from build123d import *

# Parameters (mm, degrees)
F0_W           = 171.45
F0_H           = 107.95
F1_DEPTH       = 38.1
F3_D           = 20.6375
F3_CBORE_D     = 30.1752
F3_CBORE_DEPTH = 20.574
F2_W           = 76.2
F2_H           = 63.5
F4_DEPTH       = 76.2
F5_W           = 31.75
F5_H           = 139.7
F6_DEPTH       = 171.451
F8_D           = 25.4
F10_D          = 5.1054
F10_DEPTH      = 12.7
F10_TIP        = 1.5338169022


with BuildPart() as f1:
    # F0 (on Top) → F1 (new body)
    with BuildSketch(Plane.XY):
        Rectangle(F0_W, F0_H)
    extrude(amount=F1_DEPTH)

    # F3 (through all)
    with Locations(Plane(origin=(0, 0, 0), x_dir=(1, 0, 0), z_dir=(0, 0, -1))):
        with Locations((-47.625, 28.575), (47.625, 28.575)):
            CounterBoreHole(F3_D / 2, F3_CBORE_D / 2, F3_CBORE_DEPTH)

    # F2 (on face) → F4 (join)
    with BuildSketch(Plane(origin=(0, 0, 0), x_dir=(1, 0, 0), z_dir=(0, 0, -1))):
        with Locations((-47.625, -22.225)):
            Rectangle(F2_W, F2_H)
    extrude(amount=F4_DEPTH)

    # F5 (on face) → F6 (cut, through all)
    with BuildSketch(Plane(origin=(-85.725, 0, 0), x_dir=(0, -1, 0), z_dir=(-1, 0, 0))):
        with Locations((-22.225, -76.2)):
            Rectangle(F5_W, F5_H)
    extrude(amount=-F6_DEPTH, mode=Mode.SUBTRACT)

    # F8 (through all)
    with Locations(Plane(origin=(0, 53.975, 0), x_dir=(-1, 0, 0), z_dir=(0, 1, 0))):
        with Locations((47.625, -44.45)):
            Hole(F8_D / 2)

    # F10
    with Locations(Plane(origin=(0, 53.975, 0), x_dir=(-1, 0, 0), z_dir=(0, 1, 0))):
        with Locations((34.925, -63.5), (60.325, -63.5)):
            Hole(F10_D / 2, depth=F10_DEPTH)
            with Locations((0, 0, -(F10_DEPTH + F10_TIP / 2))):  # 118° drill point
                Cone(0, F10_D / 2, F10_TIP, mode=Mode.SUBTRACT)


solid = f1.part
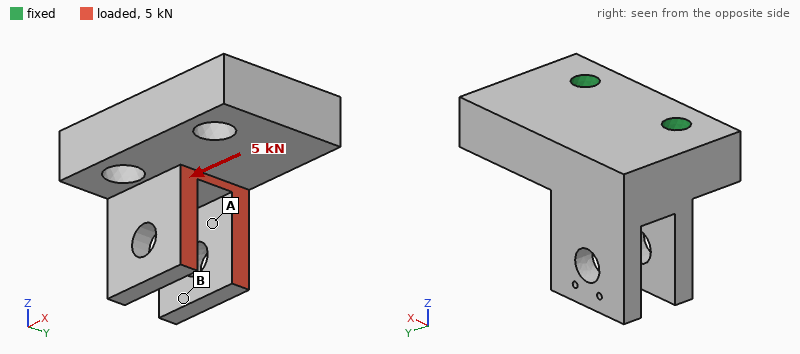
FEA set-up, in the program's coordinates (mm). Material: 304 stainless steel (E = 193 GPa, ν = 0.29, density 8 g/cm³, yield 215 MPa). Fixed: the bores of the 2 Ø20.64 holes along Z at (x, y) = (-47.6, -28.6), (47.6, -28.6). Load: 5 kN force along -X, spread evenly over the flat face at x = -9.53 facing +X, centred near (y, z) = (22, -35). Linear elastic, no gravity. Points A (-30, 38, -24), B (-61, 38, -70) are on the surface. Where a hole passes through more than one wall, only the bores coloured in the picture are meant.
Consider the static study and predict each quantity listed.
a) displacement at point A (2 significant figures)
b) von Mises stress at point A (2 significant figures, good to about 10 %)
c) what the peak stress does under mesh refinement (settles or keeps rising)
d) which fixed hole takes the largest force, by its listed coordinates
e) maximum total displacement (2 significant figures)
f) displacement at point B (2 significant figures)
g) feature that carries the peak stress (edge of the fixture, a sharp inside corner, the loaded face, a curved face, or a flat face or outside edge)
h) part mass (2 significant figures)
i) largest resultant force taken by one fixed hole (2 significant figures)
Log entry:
5.9 µm
3.8 MPa
keeps rising
(47.6, -28.6)
15 µm
13 µm
edge of the fixture
6.8 kg
5.1 kN
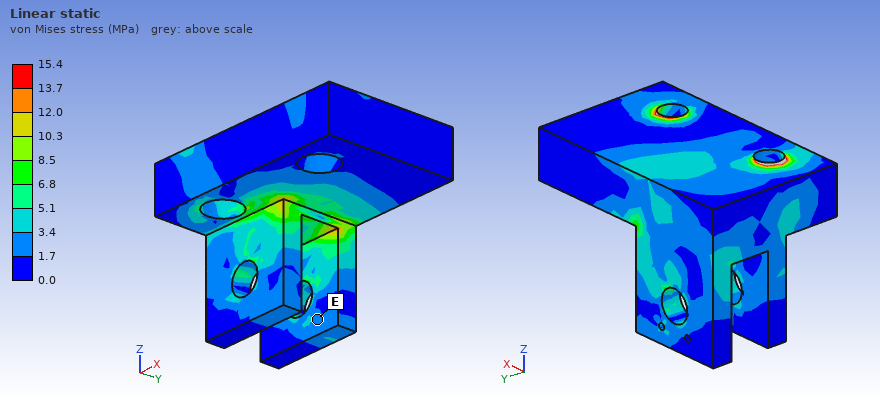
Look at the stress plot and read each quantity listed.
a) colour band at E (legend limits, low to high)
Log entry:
1.7 to 3.4 MPa
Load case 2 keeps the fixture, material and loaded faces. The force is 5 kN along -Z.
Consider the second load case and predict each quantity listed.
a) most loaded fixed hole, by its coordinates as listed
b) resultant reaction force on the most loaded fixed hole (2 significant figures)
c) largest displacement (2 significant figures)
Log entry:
(-47.6, -28.6)
3.2 kN
24 µm
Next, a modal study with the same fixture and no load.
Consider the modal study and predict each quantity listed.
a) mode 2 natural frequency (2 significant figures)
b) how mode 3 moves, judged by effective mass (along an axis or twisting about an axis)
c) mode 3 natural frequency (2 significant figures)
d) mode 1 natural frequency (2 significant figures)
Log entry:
2100 Hz
along Z
2600 Hz
1300 Hz
